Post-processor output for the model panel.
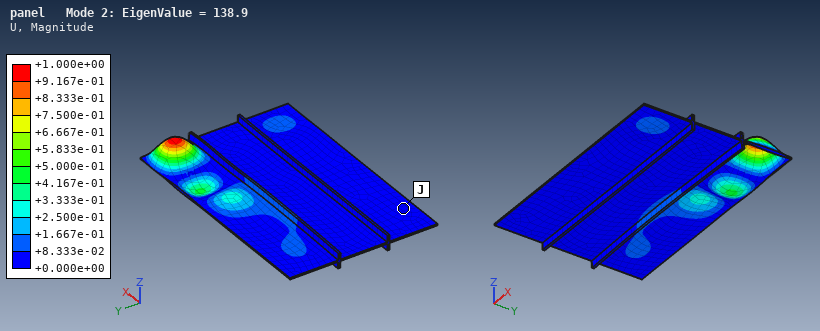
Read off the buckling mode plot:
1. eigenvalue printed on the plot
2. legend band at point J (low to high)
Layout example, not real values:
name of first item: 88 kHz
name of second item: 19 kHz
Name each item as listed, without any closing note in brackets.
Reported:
eigenvalue printed on the plot: 138.9
legend band at point J: +0.000e+00 to +8.333e-02
